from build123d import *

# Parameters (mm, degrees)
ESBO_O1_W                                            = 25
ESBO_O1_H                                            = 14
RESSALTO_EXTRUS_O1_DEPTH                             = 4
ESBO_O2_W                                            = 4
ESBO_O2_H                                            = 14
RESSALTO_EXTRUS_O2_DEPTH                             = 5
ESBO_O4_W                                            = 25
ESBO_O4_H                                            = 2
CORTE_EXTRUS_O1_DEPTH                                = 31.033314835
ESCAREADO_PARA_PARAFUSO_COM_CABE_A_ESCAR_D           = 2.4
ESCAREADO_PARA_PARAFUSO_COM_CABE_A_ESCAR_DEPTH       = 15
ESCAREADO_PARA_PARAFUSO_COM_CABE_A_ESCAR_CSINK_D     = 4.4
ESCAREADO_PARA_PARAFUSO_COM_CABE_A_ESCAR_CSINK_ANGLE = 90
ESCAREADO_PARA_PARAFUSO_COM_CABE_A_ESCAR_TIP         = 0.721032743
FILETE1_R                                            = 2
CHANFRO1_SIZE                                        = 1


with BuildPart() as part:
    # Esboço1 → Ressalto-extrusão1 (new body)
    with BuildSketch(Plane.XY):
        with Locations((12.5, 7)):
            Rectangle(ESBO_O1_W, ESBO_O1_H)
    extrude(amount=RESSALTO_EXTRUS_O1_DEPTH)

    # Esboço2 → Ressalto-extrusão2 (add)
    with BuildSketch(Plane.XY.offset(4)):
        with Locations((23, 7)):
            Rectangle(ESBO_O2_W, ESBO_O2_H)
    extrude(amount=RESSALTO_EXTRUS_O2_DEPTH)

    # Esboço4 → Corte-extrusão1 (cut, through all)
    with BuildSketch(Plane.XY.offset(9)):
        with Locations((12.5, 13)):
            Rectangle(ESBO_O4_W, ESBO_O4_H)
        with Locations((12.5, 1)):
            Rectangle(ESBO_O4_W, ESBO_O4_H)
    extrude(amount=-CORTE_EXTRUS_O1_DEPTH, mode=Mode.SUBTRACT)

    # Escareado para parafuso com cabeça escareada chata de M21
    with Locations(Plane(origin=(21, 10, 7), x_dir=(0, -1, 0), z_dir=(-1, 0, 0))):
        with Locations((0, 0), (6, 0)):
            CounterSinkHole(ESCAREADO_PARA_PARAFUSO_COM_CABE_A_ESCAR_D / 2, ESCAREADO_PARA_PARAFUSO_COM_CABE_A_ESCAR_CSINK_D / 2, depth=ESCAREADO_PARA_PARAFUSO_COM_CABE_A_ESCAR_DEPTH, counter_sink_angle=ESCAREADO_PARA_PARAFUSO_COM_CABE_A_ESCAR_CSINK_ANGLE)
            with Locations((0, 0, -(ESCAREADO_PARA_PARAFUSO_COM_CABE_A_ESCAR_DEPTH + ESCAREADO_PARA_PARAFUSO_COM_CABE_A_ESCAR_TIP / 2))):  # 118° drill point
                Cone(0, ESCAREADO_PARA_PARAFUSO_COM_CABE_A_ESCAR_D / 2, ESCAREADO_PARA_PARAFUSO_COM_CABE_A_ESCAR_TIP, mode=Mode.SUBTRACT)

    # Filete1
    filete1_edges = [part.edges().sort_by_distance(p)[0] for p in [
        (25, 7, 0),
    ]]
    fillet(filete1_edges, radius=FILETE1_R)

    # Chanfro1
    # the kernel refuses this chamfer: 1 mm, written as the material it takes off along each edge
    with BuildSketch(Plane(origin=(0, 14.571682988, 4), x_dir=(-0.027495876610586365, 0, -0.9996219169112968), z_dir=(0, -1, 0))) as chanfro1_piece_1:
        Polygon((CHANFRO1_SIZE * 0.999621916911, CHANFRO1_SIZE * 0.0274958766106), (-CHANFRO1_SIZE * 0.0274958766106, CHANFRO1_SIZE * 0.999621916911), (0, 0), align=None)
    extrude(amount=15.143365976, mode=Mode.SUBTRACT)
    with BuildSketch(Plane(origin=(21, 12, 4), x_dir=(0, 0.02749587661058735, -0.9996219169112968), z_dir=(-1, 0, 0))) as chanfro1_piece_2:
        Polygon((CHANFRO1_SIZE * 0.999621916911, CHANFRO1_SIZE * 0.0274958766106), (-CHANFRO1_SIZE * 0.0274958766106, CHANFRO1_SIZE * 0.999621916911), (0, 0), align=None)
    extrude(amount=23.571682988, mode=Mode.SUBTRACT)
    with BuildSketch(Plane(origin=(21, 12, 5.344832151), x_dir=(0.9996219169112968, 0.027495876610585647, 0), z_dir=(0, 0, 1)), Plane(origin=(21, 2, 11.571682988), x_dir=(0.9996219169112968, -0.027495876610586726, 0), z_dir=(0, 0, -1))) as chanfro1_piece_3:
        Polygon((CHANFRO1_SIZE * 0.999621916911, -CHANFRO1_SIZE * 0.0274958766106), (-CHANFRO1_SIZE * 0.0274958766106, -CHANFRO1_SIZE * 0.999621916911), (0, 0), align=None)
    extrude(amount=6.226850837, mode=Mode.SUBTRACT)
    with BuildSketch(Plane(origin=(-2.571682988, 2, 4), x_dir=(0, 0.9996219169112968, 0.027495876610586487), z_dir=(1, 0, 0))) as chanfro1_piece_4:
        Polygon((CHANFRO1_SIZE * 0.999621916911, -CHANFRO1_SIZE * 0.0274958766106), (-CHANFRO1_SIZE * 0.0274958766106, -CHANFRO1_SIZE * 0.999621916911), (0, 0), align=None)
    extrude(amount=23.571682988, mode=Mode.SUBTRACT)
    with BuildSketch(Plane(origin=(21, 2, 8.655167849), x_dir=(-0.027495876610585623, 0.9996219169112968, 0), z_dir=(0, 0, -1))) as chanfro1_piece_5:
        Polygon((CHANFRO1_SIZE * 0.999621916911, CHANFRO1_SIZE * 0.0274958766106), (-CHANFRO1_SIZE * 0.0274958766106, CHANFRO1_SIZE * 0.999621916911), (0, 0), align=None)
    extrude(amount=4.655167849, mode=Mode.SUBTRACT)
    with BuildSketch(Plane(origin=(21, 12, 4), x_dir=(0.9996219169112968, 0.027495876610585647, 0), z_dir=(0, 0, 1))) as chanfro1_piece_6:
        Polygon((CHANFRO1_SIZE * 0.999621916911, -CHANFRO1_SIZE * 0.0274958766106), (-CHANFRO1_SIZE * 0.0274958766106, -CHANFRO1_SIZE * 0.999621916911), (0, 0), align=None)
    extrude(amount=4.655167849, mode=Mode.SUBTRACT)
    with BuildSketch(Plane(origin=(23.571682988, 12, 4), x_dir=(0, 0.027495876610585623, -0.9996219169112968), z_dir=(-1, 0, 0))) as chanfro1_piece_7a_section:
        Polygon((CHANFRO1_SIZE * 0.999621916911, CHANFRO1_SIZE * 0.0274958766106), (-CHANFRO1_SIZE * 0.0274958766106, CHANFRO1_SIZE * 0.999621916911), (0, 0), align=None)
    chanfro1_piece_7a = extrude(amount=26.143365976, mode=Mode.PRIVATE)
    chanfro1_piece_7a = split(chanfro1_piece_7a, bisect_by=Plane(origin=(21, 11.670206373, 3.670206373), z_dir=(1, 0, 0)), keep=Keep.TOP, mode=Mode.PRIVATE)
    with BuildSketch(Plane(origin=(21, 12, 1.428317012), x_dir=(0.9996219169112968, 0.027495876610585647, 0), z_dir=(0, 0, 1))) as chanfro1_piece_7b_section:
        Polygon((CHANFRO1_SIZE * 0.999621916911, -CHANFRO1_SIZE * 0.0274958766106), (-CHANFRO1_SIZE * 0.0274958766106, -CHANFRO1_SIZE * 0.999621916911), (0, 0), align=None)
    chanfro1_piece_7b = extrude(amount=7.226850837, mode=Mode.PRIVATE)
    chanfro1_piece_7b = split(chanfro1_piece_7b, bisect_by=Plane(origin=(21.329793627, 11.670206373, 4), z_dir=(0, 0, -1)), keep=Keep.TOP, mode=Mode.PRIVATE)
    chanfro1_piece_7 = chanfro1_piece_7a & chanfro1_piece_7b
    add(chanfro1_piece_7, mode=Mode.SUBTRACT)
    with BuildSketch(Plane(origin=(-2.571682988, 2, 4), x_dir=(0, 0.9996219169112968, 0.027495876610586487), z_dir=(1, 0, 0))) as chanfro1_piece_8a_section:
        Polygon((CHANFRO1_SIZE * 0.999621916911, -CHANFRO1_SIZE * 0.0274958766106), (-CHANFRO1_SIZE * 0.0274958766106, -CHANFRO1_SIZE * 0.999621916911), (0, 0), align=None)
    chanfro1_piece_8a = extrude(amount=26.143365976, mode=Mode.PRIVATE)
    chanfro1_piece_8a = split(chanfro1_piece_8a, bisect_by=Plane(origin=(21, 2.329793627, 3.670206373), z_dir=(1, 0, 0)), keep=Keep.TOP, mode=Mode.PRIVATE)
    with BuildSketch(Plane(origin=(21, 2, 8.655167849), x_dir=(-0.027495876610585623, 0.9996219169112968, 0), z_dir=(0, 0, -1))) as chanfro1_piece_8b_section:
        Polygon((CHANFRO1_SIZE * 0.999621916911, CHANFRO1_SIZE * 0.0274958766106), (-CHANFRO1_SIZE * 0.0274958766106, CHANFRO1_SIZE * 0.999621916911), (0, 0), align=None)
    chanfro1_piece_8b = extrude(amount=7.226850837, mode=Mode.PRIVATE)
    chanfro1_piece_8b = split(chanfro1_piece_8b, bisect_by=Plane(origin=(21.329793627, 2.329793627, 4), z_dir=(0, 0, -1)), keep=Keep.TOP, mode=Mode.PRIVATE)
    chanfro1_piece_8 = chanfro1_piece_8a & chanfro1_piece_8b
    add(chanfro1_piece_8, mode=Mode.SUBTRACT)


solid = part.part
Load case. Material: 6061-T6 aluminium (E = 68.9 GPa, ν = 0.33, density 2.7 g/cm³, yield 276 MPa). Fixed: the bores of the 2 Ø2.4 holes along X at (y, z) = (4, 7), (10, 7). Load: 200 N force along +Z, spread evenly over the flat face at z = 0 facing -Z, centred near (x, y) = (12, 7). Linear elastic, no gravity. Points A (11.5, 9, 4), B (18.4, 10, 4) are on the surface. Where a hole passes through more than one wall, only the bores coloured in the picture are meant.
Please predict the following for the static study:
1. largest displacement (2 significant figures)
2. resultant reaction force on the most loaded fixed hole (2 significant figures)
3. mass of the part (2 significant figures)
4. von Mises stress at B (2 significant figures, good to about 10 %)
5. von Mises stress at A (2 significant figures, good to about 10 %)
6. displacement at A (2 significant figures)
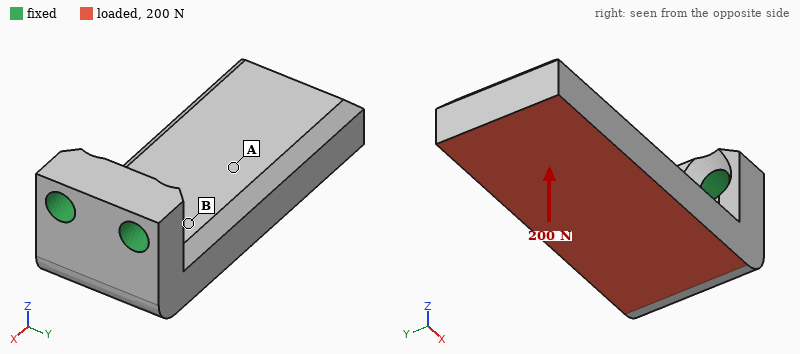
0.15 mm
110 N
3.0 g
56 MPa
23 MPa
0.063 mm
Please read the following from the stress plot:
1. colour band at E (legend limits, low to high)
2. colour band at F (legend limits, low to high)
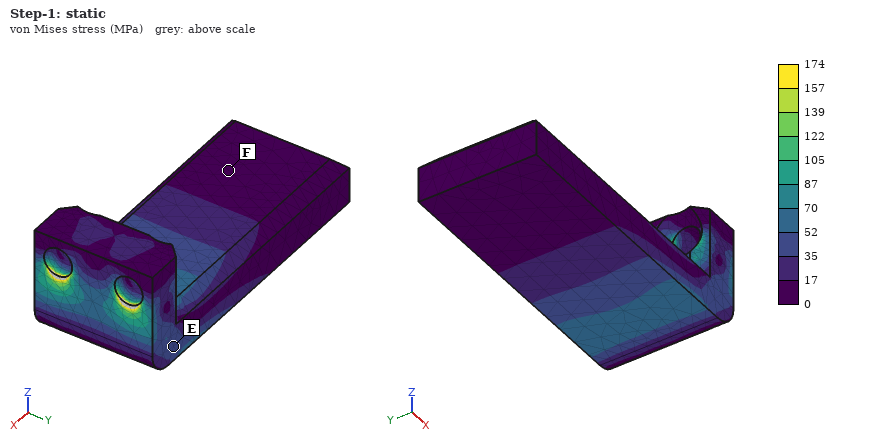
35 to 52 MPa
0 to 17 MPa
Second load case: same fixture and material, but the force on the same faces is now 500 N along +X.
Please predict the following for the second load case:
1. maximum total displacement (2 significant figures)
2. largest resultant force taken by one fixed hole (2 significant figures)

0.13 mm
250 N
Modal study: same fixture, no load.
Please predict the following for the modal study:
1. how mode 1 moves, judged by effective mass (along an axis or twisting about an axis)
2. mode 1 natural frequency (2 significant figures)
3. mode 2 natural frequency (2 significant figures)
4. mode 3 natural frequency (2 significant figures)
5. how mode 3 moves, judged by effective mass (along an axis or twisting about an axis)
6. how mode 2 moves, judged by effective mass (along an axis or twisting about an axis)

along Z
4600 Hz
8200 Hz
23 kHz
twisting about X
along Y
